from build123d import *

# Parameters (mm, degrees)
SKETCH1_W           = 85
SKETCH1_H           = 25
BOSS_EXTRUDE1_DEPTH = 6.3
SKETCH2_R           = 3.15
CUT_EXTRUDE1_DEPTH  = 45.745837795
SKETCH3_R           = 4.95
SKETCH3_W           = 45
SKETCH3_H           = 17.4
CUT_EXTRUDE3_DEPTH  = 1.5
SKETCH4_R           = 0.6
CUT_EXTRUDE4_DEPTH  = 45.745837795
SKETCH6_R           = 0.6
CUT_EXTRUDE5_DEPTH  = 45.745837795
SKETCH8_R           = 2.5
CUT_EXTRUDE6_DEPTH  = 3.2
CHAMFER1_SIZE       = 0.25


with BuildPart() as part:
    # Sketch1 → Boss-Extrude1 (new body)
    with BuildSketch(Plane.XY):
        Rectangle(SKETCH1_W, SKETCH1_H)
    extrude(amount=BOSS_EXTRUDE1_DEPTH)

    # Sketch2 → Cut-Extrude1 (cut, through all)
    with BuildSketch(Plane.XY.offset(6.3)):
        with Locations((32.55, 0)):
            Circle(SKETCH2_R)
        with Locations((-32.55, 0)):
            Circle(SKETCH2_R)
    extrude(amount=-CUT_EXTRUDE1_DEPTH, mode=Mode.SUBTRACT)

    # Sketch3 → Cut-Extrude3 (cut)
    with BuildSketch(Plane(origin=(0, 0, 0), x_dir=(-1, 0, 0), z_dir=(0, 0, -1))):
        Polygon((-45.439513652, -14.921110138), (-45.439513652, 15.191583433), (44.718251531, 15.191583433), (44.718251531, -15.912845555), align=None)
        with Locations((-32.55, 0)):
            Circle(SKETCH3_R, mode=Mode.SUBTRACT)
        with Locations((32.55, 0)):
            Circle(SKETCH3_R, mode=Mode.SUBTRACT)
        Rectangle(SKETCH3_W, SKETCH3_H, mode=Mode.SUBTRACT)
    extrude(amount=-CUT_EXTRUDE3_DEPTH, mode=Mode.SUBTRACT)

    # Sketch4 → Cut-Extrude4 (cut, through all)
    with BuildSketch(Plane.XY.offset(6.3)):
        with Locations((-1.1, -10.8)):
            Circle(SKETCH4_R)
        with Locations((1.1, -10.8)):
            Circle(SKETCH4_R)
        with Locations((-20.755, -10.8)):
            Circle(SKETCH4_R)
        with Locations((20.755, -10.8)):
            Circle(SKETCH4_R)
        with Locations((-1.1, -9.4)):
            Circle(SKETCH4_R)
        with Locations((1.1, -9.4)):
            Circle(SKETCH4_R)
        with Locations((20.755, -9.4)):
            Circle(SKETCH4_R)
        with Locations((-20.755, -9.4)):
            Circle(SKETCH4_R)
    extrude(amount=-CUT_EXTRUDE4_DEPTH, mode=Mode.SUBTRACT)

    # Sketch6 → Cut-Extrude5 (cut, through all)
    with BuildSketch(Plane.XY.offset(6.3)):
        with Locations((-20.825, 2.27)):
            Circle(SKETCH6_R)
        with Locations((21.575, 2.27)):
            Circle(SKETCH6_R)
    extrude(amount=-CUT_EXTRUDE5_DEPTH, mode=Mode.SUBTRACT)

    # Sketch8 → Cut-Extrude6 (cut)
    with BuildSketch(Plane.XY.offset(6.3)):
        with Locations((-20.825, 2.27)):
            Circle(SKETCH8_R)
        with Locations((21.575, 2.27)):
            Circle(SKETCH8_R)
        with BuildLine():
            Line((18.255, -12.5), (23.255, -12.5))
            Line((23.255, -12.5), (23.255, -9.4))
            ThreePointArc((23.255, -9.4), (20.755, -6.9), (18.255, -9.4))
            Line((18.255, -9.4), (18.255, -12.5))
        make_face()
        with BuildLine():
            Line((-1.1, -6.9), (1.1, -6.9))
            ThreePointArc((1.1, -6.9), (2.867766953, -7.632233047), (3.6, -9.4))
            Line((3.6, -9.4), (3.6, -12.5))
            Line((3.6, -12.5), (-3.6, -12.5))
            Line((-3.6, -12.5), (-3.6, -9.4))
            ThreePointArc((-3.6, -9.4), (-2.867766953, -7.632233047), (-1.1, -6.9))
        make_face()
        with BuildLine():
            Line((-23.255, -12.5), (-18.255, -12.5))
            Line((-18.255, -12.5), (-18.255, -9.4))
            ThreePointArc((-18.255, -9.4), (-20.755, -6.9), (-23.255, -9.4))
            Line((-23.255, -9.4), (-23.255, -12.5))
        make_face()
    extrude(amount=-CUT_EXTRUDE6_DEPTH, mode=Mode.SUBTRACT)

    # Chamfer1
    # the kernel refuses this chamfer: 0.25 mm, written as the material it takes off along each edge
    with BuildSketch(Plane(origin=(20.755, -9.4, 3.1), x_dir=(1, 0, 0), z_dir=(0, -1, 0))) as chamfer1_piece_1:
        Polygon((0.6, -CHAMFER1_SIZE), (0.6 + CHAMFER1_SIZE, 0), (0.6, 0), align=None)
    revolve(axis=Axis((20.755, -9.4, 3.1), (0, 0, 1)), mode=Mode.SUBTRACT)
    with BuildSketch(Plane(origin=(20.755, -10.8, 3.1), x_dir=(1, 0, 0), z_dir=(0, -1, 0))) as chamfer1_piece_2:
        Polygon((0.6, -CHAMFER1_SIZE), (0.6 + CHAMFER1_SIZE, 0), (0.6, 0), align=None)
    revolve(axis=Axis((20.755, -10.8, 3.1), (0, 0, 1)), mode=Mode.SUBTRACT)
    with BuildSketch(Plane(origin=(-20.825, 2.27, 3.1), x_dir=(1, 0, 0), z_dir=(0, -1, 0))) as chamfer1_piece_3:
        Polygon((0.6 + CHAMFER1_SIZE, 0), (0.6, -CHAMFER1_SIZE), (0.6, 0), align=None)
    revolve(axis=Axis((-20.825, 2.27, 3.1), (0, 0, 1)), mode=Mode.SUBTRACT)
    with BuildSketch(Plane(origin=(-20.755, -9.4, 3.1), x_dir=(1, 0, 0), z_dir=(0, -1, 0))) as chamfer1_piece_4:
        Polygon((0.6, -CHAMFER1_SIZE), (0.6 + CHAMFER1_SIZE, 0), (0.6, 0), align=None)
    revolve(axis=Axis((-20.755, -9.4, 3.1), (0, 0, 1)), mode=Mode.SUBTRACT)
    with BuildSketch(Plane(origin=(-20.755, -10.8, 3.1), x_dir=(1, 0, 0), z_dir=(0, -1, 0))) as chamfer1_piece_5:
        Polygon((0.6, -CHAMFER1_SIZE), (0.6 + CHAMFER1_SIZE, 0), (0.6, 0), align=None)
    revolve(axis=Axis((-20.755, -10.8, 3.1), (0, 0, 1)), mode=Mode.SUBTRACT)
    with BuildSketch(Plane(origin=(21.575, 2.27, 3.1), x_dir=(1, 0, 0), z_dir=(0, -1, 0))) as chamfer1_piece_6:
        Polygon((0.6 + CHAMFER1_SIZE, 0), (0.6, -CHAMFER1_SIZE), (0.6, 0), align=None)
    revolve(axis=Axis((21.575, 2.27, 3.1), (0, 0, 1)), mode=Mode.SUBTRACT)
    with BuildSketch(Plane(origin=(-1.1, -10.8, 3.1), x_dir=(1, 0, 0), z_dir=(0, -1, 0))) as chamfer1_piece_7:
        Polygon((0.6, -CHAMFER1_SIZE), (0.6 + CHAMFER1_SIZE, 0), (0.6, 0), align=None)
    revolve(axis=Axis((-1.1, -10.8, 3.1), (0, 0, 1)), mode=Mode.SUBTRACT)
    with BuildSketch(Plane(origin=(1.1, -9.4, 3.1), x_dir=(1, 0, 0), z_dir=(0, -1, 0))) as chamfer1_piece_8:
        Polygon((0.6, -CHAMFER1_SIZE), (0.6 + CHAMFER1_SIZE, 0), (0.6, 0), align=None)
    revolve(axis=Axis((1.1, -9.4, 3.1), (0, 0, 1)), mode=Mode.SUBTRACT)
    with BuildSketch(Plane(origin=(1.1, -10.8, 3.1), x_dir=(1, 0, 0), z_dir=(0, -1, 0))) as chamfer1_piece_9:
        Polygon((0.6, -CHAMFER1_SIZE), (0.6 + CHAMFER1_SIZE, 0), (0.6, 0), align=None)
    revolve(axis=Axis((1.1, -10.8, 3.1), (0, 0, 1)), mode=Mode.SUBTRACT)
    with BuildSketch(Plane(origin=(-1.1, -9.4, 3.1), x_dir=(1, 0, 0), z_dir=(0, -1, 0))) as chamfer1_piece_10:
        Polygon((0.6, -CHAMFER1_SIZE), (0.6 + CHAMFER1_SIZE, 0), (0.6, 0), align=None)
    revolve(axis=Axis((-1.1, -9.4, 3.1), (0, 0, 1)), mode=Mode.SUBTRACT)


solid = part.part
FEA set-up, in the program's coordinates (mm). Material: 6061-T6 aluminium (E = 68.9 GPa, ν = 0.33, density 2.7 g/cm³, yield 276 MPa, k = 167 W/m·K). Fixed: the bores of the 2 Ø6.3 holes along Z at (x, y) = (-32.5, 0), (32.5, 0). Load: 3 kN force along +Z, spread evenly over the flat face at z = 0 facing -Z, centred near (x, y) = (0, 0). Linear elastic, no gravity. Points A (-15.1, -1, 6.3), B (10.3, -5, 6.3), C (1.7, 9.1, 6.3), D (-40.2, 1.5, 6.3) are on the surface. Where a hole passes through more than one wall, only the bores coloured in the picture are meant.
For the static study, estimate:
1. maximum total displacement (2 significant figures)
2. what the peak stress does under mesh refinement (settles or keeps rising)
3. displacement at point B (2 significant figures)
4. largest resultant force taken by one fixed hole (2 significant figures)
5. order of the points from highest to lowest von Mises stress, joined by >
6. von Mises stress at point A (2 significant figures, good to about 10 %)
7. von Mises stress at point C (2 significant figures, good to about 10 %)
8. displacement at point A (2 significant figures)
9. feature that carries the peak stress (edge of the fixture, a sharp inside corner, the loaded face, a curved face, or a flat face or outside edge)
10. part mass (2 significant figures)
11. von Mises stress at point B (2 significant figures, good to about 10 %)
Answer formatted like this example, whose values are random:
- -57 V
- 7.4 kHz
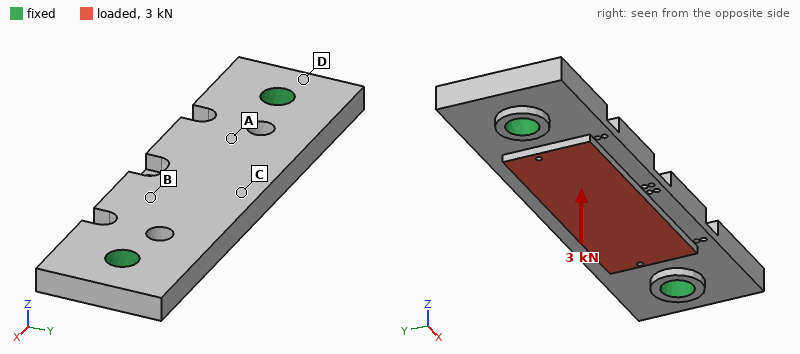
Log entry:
- 0.15 mm
- keeps rising
- 0.11 mm
- 1.7 kN
- C > B > A > D
- 37 MPa
- 83 MPa
- 0.082 mm
- edge of the fixture
- 29 g
- 61 MPa
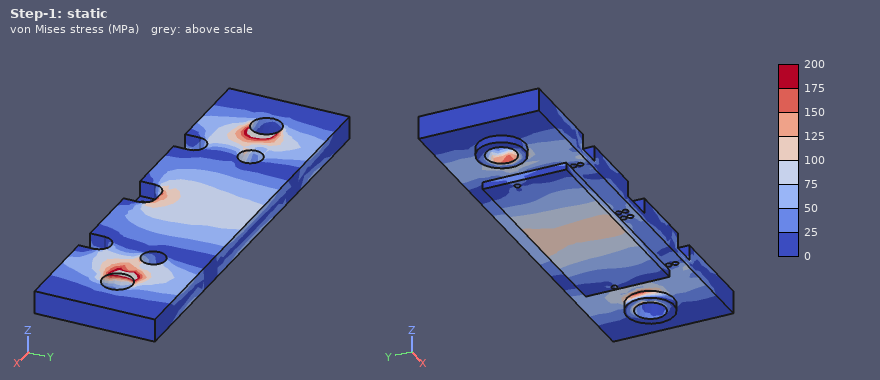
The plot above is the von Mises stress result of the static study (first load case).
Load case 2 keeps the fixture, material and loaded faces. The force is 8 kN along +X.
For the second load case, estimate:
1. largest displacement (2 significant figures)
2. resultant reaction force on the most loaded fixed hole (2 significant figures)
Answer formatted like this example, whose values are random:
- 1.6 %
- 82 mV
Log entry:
- 15 µm
- 4.0 kN
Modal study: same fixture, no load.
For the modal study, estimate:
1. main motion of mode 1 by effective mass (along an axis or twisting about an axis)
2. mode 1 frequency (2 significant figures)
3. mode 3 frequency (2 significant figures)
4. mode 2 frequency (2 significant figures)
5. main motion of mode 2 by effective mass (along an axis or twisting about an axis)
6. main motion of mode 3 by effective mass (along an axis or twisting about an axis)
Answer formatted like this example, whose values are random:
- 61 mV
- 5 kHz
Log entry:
- along Z
- 6400 Hz
- 13 kHz
- 9900 Hz
- twisting about X
- along Y
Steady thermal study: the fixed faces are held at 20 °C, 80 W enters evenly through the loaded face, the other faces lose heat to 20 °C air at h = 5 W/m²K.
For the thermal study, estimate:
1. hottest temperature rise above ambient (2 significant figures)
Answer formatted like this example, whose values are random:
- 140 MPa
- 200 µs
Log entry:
- 45 K
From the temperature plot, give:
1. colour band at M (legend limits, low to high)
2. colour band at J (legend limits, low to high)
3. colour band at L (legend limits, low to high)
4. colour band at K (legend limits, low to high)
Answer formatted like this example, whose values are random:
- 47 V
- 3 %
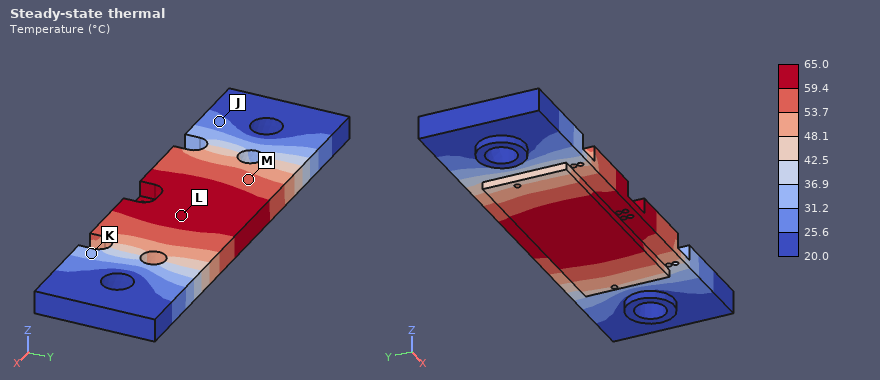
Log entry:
- 53.7 to 59.4 °C
- 25.6 to 31.2 °C
- 59.4 to 65.0 °C
- 31.2 to 36.9 °C
